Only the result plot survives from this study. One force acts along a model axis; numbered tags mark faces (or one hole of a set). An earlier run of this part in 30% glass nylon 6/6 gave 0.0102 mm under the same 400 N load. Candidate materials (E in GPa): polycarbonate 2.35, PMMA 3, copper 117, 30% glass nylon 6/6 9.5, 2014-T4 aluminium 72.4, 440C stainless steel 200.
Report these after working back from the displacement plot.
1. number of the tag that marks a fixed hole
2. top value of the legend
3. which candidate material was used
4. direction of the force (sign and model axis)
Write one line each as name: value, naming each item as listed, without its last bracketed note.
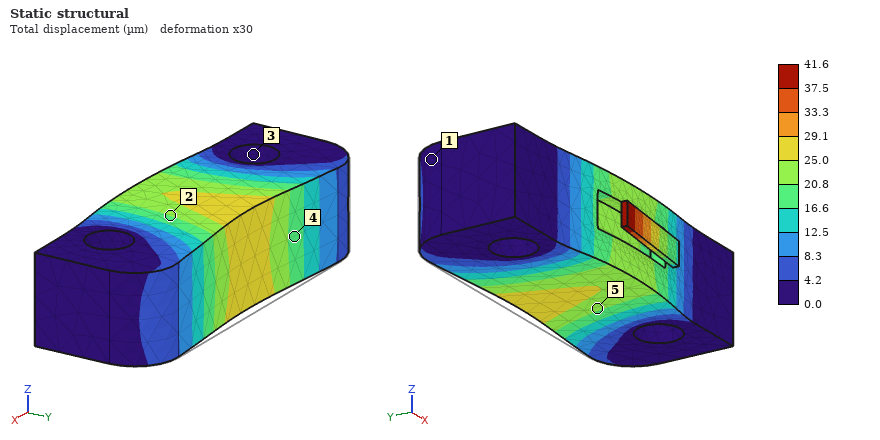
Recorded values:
number of the tag that marks a fixed hole: 3
top value of the legend: 41.6 µm
which candidate material was used: polycarbonate
direction of the force: -Y
